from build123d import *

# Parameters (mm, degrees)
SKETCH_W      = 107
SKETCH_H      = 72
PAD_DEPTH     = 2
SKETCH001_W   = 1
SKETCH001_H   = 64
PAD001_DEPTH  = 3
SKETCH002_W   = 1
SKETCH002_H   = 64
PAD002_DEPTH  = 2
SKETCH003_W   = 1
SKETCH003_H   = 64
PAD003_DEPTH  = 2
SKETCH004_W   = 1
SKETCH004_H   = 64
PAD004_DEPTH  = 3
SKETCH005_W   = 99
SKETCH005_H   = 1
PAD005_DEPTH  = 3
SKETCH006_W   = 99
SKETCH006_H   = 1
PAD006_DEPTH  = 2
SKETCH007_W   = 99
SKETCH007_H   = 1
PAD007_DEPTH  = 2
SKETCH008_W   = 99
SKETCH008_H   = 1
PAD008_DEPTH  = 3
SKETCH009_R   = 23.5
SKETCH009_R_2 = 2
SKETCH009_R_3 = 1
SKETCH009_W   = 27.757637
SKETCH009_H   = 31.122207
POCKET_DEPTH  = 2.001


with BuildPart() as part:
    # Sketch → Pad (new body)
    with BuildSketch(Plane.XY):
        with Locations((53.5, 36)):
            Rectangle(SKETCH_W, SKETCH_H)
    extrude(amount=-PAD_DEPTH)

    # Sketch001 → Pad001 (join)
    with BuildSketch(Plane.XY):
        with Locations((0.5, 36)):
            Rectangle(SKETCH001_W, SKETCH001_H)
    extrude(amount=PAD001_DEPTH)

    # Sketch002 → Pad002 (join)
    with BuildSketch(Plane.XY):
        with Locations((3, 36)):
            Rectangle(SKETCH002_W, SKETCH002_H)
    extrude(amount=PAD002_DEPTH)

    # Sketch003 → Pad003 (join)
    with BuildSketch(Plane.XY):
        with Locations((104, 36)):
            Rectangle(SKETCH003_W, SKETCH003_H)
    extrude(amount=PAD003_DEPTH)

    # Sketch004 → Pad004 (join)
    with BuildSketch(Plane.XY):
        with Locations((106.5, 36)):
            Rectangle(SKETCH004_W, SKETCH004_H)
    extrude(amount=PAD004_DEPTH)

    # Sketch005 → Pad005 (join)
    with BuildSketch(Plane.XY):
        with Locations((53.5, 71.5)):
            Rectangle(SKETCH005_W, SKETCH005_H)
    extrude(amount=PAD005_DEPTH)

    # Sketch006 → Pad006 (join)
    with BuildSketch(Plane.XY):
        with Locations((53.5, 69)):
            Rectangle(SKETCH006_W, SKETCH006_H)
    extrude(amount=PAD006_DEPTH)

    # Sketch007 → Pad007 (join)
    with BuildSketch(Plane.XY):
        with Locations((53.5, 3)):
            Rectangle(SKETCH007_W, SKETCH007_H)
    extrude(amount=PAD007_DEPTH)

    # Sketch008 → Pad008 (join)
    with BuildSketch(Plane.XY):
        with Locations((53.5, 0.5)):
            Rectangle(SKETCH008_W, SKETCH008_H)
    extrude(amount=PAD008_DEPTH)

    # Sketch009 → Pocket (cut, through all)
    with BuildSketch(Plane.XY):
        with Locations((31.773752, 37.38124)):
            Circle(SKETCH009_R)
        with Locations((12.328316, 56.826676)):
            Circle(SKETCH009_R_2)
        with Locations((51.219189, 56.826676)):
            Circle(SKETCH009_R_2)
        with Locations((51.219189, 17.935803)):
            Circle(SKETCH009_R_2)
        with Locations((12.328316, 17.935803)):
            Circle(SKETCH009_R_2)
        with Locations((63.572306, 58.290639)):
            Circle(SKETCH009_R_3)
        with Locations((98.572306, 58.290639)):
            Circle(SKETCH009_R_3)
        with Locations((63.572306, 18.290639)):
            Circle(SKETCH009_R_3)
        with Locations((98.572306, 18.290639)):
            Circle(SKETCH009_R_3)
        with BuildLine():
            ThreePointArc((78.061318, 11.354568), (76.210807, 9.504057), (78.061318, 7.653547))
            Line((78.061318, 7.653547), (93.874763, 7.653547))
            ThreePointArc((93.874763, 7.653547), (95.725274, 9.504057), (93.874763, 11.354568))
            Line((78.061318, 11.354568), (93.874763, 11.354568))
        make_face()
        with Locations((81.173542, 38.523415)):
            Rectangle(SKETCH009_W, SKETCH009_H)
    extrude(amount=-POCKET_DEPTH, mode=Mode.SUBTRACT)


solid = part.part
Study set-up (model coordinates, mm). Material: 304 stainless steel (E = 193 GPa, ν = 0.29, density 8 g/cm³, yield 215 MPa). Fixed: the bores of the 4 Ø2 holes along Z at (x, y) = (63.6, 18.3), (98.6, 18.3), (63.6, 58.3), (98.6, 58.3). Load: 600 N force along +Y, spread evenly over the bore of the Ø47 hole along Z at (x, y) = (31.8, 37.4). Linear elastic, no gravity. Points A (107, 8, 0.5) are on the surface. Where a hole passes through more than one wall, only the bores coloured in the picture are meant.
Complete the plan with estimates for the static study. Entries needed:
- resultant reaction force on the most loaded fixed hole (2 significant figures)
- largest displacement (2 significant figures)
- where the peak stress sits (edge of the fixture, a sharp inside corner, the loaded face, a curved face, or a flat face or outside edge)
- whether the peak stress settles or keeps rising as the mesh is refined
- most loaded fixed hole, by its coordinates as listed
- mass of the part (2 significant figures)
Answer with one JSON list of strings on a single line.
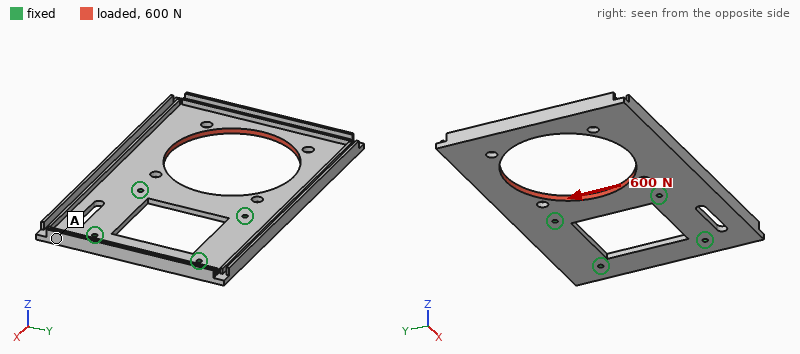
["450 N", "42 µm", "edge of the fixture", "keeps rising", "(63.6, 18.3)", "93 g"]
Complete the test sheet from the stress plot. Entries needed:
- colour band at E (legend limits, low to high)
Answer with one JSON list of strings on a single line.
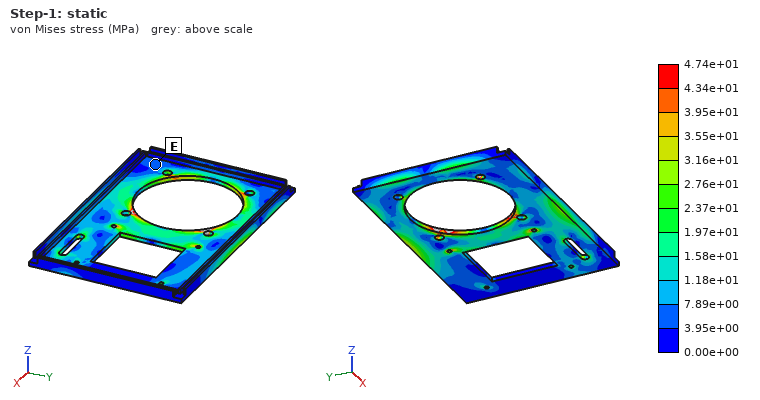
["3.95e+00 to 7.89e+00 MPa"]
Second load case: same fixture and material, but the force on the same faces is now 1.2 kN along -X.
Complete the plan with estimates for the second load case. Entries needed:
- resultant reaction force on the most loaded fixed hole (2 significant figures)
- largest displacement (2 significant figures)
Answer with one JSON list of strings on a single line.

["460 N", "31 µm"]
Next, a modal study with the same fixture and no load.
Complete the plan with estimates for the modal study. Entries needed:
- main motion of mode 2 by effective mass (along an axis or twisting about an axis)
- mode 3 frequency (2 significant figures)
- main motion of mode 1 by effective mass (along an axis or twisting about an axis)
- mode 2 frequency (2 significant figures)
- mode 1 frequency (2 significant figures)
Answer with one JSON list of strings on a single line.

["twisting about X", "2300 Hz", "along Z", "720 Hz", "430 Hz"]
